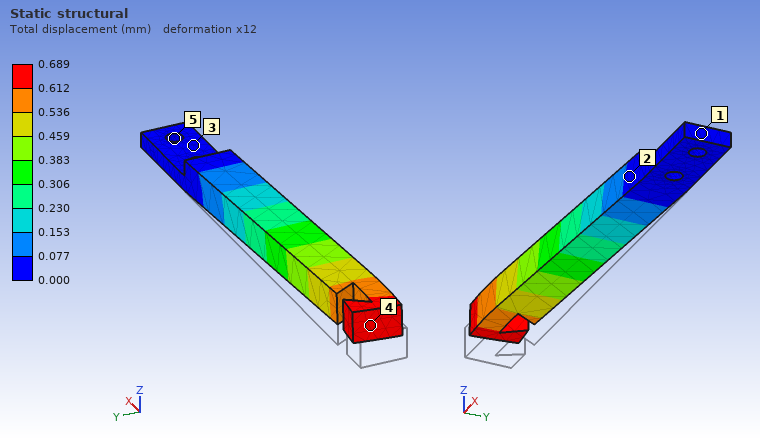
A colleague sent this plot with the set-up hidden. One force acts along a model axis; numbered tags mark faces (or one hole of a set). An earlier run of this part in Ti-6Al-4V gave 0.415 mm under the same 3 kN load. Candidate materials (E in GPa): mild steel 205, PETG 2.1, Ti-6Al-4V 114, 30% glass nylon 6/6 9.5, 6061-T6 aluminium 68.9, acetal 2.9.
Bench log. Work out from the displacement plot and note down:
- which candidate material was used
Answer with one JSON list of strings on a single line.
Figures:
["6061-T6 aluminium"]
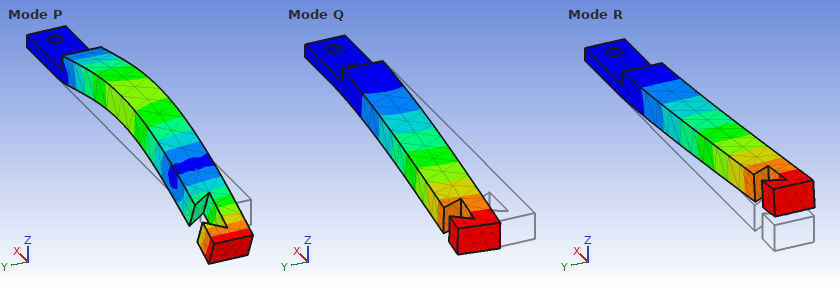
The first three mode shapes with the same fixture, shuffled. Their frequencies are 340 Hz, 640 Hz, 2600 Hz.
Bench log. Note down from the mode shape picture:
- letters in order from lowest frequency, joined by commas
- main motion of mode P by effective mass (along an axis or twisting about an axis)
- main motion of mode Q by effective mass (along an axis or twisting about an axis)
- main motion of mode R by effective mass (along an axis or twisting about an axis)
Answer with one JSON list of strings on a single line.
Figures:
["R, Q, P", "along Z", "along Y", "along Z"]
